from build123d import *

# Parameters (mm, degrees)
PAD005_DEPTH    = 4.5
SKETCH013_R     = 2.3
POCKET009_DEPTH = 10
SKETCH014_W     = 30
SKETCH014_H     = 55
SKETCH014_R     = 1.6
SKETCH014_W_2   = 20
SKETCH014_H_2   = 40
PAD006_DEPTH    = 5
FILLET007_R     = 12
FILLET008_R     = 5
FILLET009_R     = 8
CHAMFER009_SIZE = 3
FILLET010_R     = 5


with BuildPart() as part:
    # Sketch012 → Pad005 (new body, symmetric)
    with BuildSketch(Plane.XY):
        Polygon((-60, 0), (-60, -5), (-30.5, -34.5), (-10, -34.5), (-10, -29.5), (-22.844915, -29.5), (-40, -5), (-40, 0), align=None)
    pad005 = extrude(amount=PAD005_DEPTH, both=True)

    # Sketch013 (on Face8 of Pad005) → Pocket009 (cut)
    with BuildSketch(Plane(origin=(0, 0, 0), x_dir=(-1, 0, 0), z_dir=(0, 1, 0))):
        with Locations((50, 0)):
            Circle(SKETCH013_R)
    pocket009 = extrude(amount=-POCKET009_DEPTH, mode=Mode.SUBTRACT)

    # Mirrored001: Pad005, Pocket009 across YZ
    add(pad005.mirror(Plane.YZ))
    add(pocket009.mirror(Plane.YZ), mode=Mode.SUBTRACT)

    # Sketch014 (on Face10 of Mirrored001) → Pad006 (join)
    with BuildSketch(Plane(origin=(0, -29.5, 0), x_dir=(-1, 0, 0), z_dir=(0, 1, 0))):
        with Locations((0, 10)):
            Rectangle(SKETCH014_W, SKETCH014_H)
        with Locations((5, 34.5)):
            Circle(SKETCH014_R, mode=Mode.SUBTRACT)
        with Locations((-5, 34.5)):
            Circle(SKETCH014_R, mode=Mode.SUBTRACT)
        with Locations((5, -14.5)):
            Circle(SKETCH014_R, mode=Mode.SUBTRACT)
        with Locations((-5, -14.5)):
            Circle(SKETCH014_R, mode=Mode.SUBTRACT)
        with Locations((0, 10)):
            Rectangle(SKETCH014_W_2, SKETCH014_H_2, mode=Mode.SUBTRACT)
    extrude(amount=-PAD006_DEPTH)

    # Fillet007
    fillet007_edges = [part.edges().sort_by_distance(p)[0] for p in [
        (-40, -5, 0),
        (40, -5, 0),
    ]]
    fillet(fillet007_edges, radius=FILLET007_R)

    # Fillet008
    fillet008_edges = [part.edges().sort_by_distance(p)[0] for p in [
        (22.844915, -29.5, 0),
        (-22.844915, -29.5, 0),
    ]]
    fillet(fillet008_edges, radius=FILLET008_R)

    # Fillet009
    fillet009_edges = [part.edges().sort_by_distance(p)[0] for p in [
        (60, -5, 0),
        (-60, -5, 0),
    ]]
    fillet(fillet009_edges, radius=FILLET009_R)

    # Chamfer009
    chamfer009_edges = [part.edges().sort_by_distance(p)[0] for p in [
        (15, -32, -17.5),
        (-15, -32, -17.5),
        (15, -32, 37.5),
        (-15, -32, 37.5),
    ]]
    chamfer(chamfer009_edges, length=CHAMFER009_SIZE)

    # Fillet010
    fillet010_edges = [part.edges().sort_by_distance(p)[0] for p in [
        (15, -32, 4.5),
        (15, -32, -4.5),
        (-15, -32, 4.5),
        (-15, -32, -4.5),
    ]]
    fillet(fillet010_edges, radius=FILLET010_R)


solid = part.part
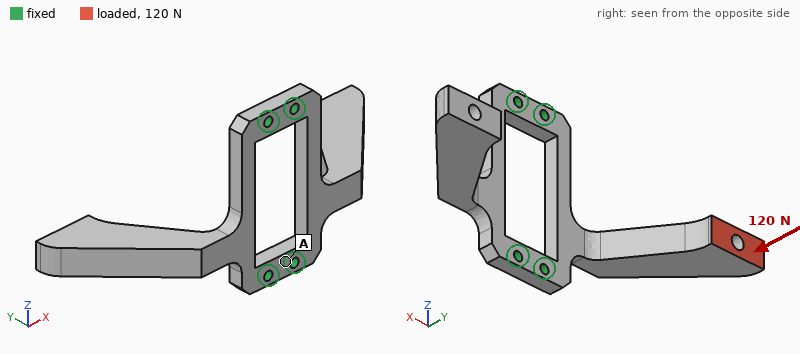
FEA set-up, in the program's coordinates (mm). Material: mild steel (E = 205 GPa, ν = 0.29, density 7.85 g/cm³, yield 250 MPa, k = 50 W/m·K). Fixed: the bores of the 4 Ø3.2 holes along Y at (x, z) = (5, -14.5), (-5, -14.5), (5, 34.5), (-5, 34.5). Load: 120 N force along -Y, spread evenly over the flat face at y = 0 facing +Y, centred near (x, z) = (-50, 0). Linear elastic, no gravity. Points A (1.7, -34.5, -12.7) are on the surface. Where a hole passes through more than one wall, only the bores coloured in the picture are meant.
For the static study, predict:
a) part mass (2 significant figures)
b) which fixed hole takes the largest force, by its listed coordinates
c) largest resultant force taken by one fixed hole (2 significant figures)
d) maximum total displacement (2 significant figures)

110 g
(-5, -14.5)
130 N
0.38 mm
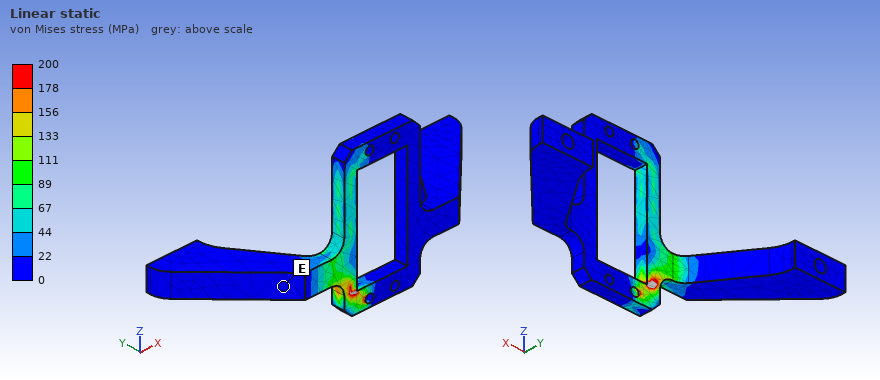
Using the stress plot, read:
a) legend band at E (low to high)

0 to 22 MPa
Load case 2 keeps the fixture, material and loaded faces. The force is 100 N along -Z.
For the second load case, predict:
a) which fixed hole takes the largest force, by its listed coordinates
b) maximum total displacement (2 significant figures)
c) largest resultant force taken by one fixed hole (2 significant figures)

(-5, 34.5)
0.14 mm
160 N
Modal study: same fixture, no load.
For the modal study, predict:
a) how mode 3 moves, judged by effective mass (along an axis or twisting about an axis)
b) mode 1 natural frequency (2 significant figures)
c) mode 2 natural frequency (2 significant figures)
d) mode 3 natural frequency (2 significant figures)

along Z
610 Hz
610 Hz
1200 Hz
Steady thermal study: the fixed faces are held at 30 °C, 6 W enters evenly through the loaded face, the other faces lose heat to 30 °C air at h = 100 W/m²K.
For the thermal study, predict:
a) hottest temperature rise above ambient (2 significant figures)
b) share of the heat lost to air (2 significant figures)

35 K
86 %
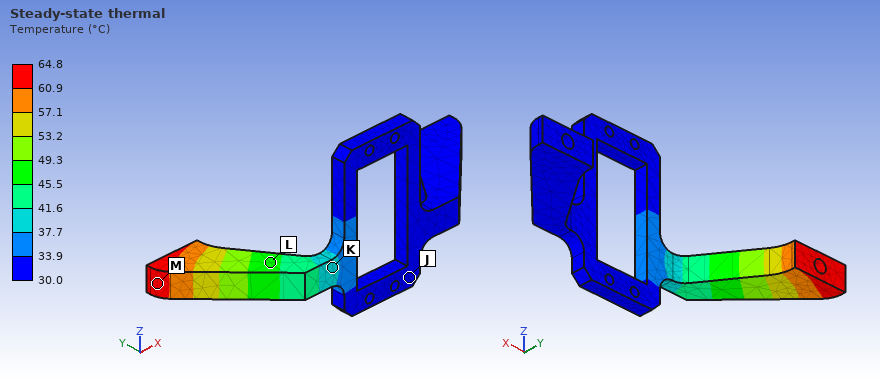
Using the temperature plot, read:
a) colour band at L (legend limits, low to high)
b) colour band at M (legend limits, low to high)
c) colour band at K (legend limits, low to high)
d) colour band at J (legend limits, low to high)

45.5 to 49.3 °C
60.9 to 64.8 °C
37.7 to 41.6 °C
30.0 to 33.9 °C
